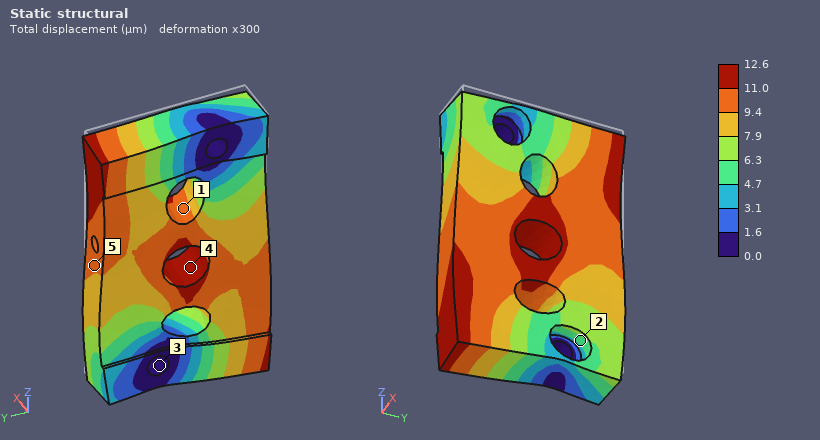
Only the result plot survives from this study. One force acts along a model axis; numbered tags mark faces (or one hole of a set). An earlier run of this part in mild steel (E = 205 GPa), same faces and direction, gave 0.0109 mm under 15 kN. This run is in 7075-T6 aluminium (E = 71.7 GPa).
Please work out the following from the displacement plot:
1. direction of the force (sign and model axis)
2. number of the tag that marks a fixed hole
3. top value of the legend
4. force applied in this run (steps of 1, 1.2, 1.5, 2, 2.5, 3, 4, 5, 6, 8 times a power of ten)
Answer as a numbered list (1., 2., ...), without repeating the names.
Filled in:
1. -Z
2. 3
3. 12.6 µm
4. 6 kN
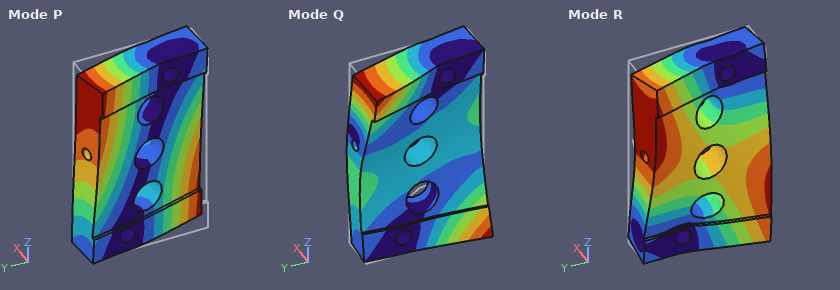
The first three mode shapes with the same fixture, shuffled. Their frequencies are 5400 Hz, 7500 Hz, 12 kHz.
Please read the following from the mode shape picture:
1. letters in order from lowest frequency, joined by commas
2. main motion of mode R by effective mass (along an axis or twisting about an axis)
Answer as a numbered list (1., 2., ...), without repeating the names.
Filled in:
1. P, R, Q
2. along X
